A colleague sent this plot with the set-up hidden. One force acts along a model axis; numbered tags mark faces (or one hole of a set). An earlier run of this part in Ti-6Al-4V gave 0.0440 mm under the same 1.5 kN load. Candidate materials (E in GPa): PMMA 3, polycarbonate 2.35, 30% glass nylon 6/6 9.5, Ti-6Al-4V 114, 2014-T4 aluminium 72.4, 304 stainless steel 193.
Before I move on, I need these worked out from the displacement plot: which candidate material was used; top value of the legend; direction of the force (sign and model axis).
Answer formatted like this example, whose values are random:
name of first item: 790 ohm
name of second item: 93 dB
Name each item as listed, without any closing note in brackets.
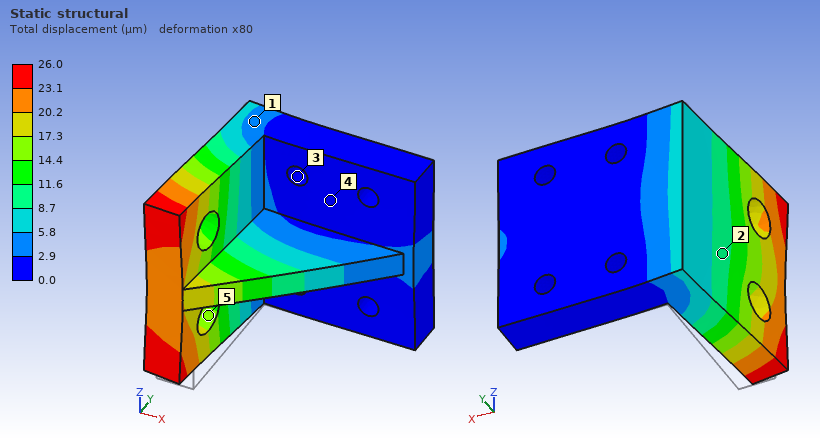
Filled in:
which candidate material was used: 304 stainless steel
top value of the legend: 26.0 µm
direction of the force: -X
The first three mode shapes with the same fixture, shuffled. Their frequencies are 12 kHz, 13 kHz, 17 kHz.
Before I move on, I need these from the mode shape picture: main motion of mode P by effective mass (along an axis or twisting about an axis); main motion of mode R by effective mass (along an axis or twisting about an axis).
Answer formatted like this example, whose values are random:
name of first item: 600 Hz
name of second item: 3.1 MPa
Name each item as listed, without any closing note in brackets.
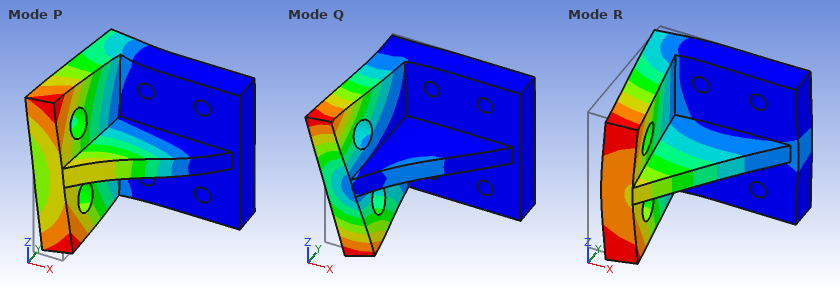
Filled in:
main motion of mode P by effective mass: along Z
main motion of mode R by effective mass: along X
